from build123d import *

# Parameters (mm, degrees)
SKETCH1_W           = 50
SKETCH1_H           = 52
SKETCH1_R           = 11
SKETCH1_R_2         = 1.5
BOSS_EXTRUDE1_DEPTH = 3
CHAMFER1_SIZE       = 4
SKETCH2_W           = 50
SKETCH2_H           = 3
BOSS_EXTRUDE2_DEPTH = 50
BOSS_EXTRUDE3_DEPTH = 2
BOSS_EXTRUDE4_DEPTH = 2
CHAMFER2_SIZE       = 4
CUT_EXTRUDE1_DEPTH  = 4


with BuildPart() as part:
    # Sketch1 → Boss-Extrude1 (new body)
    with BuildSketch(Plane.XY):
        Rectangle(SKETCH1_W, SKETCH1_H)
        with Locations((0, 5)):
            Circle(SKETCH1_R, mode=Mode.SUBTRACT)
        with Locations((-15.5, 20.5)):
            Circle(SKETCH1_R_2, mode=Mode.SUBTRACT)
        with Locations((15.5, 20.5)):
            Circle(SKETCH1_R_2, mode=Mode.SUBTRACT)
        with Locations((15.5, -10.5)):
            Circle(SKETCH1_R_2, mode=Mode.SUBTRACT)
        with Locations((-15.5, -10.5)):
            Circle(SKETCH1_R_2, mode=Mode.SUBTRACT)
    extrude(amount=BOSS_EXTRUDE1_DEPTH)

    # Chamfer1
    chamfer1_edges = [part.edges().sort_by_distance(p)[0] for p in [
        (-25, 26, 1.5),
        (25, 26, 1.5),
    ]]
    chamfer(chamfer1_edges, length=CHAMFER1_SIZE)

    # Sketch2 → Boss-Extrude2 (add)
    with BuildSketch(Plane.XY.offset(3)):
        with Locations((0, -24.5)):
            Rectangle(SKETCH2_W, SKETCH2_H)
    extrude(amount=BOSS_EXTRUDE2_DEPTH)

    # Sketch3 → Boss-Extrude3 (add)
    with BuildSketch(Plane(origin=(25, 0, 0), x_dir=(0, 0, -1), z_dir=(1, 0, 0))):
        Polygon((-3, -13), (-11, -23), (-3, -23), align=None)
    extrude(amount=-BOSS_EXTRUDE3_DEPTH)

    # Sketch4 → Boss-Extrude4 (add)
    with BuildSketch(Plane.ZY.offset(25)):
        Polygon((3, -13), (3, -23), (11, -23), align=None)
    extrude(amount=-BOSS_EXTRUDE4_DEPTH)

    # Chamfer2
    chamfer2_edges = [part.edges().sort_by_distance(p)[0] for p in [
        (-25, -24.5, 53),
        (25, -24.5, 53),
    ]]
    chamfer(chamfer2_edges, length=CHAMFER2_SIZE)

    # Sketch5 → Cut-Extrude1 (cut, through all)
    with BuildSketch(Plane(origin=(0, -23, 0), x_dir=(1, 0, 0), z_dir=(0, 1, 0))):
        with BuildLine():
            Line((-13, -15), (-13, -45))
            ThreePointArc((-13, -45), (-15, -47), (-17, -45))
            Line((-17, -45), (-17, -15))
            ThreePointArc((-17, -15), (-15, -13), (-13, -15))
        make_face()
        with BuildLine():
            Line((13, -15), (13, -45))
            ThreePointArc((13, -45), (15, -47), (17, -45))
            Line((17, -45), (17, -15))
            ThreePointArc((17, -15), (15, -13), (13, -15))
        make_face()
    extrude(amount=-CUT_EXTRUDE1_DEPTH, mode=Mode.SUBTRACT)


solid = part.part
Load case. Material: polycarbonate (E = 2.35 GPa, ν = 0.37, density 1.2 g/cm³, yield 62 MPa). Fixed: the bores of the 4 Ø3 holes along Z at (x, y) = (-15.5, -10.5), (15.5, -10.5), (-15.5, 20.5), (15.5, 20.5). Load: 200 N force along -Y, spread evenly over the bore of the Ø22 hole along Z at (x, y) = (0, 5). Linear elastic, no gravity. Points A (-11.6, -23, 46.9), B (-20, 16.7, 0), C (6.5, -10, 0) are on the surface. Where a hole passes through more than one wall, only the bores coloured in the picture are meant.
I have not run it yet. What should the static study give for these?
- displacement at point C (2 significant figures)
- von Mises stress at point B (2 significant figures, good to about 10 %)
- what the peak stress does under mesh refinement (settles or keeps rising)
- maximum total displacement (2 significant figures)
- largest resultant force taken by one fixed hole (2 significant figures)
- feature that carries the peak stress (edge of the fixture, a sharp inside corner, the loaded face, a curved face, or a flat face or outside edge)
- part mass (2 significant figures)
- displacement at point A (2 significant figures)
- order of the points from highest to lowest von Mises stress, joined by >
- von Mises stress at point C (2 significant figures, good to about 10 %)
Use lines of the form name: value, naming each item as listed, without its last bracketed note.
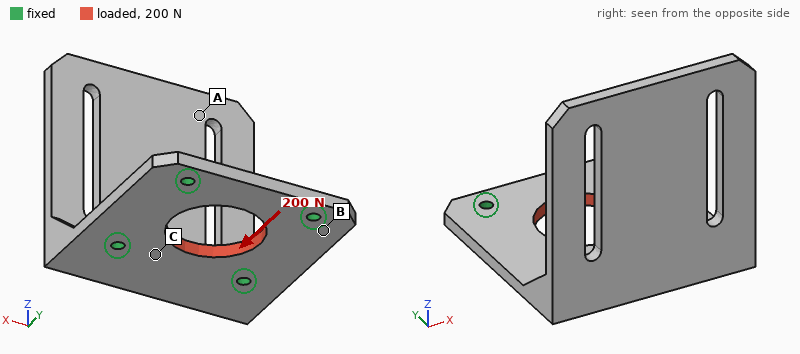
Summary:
displacement at point C: 7.1 µm
von Mises stress at point B: 0.47 MPa
what the peak stress does under mesh refinement: keeps rising
maximum total displacement: 19 µm
largest resultant force taken by one fixed hole: 52 N
feature that carries the peak stress: edge of the fixture
part mass: 16 g
displacement at point A: 7.1 µm
order of the points from highest to lowest von Mises stress, joined by >: C > B > A
von Mises stress at point C: 0.75 MPa
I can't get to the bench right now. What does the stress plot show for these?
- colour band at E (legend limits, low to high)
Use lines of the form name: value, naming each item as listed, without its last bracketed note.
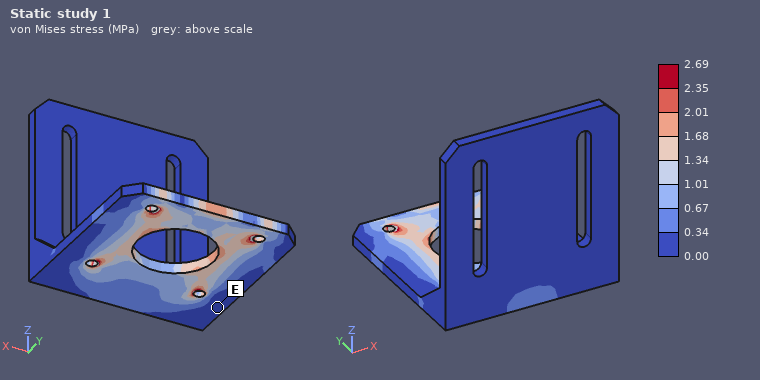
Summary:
colour band at E: 0.00 to 0.34 MPa
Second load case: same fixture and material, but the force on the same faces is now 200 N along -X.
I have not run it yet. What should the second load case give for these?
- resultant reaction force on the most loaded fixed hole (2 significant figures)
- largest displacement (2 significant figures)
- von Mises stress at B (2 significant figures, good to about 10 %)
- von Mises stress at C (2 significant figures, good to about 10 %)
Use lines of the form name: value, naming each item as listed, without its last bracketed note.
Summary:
resultant reaction force on the most loaded fixed hole: 52 N
largest displacement: 14 µm
von Mises stress at B: 0.96 MPa
von Mises stress at C: 1.1 MPa
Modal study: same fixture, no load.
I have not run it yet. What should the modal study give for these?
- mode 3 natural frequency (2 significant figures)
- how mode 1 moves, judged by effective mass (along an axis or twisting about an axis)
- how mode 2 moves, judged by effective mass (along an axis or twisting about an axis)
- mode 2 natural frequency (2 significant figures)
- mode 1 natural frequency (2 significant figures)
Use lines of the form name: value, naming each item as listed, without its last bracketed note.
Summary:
mode 3 natural frequency: 770 Hz
how mode 1 moves, judged by effective mass: along Y
how mode 2 moves, judged by effective mass: along X
mode 2 natural frequency: 500 Hz
mode 1 natural frequency: 210 Hz
